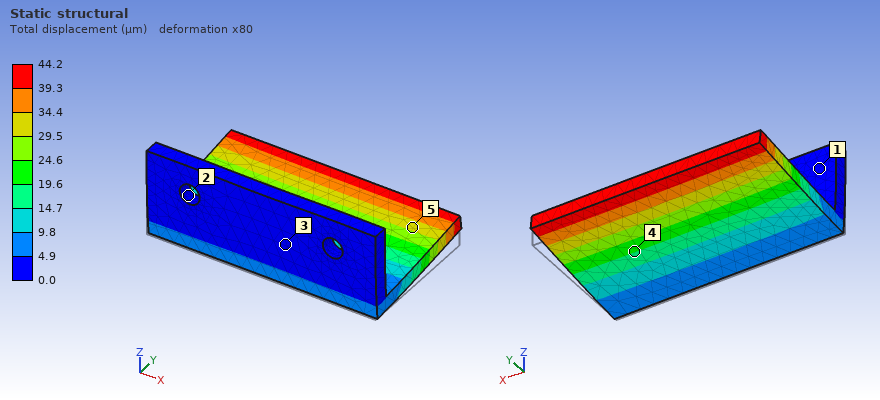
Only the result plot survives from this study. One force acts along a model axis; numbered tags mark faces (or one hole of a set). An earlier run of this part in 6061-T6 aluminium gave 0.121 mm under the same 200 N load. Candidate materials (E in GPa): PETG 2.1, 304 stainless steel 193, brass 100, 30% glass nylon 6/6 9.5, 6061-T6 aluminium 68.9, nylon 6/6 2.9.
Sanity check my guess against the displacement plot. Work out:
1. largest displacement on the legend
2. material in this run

44.2 µm
304 stainless steel
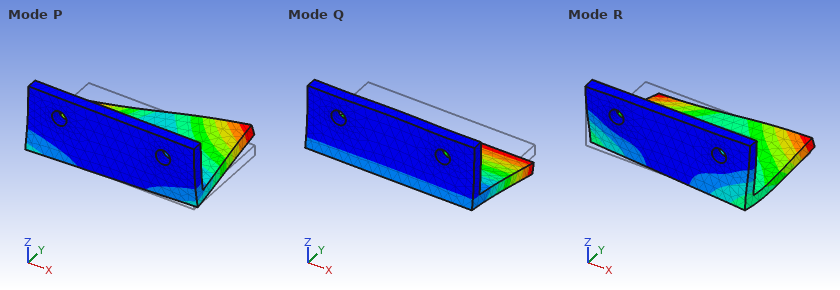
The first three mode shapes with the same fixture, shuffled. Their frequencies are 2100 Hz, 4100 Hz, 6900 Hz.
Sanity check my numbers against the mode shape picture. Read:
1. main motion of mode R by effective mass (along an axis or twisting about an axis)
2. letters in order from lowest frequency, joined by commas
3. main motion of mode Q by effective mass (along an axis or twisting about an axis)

along X
Q, P, R
along Z
